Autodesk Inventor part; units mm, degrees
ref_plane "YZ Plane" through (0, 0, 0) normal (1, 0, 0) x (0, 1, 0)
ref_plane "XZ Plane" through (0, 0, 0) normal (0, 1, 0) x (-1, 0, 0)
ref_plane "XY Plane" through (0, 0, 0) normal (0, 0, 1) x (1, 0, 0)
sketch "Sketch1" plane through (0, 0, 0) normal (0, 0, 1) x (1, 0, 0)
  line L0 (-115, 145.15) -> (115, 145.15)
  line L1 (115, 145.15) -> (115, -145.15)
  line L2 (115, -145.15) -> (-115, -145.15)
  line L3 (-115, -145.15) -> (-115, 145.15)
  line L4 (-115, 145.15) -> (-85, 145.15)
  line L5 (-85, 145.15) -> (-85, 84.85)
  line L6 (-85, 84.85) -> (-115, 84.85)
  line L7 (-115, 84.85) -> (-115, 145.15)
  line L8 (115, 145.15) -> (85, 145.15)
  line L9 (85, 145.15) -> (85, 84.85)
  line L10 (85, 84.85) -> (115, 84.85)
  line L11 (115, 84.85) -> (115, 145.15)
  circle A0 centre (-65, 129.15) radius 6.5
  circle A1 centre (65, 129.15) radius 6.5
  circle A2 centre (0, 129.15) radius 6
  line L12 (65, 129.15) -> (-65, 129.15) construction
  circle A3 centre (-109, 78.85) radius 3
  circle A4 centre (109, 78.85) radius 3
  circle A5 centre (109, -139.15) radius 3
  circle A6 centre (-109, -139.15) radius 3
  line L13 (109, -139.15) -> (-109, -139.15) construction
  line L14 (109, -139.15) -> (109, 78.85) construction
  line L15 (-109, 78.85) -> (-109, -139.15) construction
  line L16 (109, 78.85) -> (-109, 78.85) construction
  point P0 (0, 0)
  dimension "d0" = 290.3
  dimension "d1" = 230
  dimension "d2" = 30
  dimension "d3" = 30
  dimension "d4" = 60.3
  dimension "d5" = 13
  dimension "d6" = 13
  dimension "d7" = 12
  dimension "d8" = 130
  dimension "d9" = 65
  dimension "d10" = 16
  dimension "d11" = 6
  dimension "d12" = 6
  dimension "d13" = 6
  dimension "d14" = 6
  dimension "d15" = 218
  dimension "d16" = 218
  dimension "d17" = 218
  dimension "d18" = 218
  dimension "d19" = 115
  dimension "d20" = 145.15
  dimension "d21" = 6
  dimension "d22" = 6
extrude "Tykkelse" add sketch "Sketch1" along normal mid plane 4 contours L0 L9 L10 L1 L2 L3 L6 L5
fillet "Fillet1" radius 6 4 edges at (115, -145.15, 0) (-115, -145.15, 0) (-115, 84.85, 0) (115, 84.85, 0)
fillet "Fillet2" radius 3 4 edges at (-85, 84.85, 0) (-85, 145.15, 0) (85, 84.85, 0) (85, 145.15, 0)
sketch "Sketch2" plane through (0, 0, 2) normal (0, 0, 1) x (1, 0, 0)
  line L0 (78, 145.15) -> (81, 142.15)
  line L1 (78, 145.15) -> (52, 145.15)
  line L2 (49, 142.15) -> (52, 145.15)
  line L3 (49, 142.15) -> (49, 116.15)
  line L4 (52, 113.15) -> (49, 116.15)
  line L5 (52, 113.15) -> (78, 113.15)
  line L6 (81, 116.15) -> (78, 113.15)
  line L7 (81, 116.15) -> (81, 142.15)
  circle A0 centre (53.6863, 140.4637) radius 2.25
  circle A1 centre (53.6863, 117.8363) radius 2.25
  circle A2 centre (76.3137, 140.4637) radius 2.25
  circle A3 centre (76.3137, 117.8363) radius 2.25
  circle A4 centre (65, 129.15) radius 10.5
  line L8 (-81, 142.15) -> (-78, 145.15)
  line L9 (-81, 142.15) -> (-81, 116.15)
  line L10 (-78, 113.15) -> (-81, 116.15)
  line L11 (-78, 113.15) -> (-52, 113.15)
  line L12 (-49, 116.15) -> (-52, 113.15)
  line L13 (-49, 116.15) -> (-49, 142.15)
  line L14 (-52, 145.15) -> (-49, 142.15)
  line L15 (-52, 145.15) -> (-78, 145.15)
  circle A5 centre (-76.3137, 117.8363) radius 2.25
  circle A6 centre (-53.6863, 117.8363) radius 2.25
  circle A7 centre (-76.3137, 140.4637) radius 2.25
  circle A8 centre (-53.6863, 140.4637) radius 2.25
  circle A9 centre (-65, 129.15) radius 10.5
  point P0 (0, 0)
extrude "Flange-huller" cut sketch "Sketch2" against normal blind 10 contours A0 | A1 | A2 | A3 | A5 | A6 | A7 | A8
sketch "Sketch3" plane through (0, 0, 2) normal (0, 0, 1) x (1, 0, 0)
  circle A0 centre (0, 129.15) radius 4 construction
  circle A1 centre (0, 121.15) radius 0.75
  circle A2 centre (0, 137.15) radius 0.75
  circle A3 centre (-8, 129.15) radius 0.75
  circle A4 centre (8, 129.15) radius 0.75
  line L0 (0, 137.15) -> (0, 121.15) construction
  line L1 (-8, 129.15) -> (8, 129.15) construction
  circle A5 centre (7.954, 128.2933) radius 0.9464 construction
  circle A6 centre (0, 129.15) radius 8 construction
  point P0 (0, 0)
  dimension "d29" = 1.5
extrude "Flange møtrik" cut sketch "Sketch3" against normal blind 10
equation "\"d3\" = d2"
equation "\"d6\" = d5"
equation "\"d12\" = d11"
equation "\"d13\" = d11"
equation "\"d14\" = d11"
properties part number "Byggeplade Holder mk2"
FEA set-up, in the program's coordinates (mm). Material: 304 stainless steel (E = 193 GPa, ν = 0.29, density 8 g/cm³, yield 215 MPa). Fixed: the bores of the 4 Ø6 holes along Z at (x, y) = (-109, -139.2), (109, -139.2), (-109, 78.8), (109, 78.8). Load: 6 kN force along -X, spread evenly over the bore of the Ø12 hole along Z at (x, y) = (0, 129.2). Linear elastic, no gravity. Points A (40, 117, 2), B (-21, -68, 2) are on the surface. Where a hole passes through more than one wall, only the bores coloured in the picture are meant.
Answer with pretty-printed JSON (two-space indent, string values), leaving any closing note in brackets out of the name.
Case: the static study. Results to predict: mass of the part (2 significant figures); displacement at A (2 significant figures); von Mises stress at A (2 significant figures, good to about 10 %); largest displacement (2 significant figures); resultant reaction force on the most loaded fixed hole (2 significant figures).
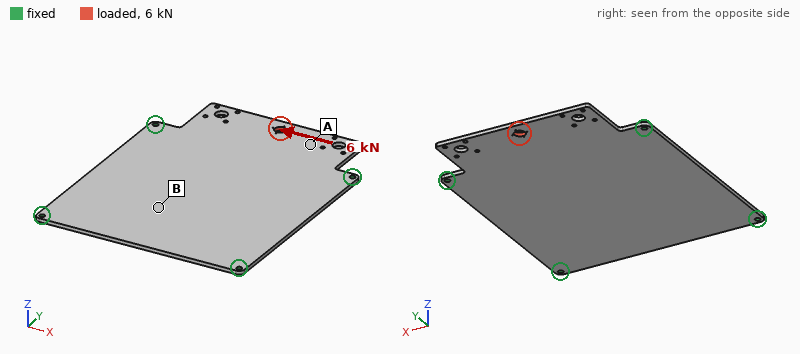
{
  "mass of the part": "2.0 kg",
  "displacement at A": "16 µm",
  "von Mises stress at A": "18 MPa",
  "largest displacement": "24 µm",
  "resultant reaction force on the most loaded fixed hole": "2.9 kN"
}
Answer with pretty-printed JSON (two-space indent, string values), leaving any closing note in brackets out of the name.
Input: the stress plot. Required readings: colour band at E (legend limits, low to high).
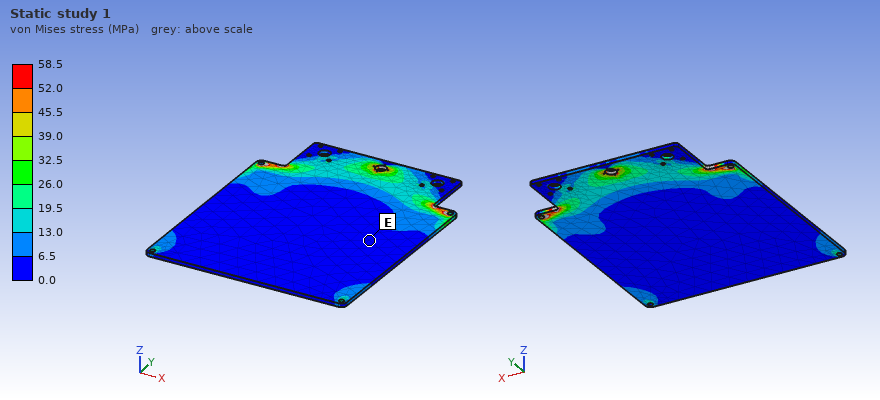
{
  "colour band at E": "0.0 to 6.5 MPa"
}
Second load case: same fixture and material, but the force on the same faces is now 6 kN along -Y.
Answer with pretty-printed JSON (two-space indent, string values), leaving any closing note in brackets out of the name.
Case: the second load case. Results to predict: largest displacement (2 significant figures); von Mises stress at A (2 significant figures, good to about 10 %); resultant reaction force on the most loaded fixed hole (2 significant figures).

{
  "largest displacement": "20 µm",
  "von Mises stress at A": "10 MPa",
  "resultant reaction force on the most loaded fixed hole": "1.7 kN"
}
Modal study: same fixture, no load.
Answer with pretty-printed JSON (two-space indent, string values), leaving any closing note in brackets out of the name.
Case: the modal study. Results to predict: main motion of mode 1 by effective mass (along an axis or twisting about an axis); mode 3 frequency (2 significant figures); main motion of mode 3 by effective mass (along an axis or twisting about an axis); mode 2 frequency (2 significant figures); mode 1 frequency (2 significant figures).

{
  "main motion of mode 1 by effective mass": "along Z",
  "mode 3 frequency": "450 Hz",
  "main motion of mode 3 by effective mass": "twisting about Y",
  "mode 2 frequency": "270 Hz",
  "mode 1 frequency": "240 Hz"
}
